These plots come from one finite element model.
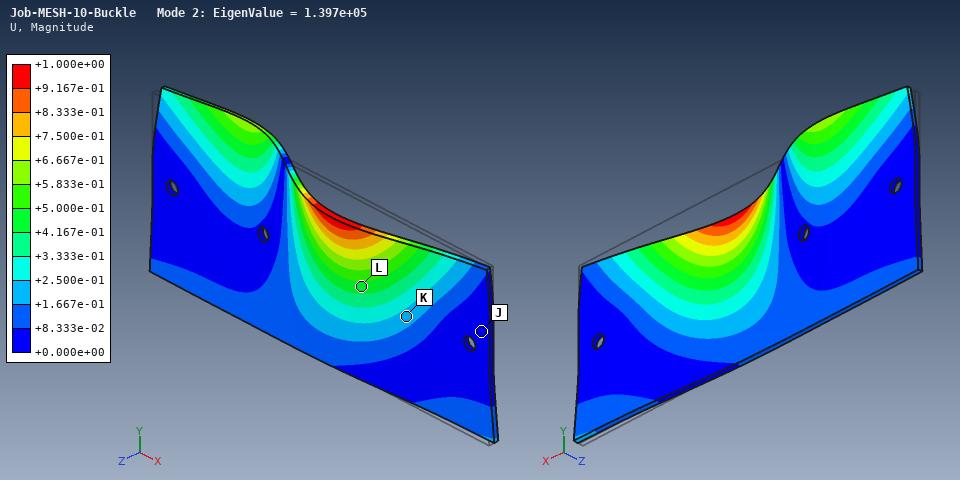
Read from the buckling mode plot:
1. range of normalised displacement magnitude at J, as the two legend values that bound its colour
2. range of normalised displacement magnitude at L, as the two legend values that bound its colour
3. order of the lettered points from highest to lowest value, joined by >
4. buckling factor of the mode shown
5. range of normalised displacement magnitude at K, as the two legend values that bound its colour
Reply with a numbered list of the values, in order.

1. +0.000e+00 to +8.333e-02
2. +4.167e-01 to +5.000e-01
3. L > K > J
4. 1.397e+05
5. +1.667e-01 to +2.500e-01
